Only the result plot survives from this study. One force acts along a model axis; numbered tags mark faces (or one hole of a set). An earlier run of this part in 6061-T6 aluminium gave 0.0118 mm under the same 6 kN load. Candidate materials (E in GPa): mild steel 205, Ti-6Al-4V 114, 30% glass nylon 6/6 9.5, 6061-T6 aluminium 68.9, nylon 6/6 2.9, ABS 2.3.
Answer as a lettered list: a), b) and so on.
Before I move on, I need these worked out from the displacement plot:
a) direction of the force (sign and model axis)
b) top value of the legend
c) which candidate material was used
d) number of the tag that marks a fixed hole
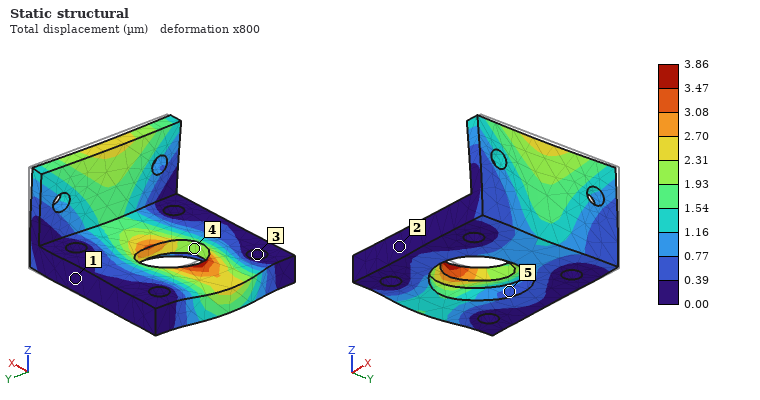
a) -X
b) 3.86 µm
c) mild steel
d) 3
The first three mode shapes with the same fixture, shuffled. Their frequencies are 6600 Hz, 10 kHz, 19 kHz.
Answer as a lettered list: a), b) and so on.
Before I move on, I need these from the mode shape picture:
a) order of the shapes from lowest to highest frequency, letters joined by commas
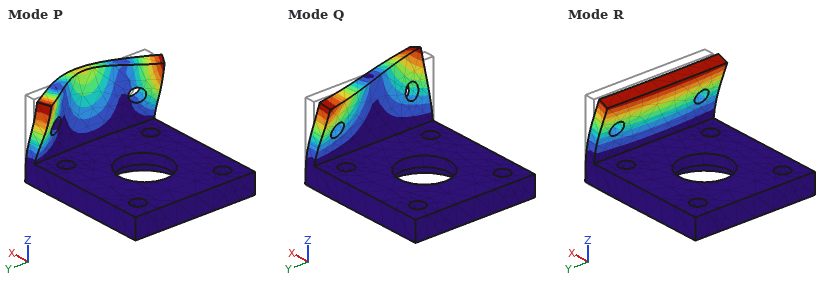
a) R, Q, P
